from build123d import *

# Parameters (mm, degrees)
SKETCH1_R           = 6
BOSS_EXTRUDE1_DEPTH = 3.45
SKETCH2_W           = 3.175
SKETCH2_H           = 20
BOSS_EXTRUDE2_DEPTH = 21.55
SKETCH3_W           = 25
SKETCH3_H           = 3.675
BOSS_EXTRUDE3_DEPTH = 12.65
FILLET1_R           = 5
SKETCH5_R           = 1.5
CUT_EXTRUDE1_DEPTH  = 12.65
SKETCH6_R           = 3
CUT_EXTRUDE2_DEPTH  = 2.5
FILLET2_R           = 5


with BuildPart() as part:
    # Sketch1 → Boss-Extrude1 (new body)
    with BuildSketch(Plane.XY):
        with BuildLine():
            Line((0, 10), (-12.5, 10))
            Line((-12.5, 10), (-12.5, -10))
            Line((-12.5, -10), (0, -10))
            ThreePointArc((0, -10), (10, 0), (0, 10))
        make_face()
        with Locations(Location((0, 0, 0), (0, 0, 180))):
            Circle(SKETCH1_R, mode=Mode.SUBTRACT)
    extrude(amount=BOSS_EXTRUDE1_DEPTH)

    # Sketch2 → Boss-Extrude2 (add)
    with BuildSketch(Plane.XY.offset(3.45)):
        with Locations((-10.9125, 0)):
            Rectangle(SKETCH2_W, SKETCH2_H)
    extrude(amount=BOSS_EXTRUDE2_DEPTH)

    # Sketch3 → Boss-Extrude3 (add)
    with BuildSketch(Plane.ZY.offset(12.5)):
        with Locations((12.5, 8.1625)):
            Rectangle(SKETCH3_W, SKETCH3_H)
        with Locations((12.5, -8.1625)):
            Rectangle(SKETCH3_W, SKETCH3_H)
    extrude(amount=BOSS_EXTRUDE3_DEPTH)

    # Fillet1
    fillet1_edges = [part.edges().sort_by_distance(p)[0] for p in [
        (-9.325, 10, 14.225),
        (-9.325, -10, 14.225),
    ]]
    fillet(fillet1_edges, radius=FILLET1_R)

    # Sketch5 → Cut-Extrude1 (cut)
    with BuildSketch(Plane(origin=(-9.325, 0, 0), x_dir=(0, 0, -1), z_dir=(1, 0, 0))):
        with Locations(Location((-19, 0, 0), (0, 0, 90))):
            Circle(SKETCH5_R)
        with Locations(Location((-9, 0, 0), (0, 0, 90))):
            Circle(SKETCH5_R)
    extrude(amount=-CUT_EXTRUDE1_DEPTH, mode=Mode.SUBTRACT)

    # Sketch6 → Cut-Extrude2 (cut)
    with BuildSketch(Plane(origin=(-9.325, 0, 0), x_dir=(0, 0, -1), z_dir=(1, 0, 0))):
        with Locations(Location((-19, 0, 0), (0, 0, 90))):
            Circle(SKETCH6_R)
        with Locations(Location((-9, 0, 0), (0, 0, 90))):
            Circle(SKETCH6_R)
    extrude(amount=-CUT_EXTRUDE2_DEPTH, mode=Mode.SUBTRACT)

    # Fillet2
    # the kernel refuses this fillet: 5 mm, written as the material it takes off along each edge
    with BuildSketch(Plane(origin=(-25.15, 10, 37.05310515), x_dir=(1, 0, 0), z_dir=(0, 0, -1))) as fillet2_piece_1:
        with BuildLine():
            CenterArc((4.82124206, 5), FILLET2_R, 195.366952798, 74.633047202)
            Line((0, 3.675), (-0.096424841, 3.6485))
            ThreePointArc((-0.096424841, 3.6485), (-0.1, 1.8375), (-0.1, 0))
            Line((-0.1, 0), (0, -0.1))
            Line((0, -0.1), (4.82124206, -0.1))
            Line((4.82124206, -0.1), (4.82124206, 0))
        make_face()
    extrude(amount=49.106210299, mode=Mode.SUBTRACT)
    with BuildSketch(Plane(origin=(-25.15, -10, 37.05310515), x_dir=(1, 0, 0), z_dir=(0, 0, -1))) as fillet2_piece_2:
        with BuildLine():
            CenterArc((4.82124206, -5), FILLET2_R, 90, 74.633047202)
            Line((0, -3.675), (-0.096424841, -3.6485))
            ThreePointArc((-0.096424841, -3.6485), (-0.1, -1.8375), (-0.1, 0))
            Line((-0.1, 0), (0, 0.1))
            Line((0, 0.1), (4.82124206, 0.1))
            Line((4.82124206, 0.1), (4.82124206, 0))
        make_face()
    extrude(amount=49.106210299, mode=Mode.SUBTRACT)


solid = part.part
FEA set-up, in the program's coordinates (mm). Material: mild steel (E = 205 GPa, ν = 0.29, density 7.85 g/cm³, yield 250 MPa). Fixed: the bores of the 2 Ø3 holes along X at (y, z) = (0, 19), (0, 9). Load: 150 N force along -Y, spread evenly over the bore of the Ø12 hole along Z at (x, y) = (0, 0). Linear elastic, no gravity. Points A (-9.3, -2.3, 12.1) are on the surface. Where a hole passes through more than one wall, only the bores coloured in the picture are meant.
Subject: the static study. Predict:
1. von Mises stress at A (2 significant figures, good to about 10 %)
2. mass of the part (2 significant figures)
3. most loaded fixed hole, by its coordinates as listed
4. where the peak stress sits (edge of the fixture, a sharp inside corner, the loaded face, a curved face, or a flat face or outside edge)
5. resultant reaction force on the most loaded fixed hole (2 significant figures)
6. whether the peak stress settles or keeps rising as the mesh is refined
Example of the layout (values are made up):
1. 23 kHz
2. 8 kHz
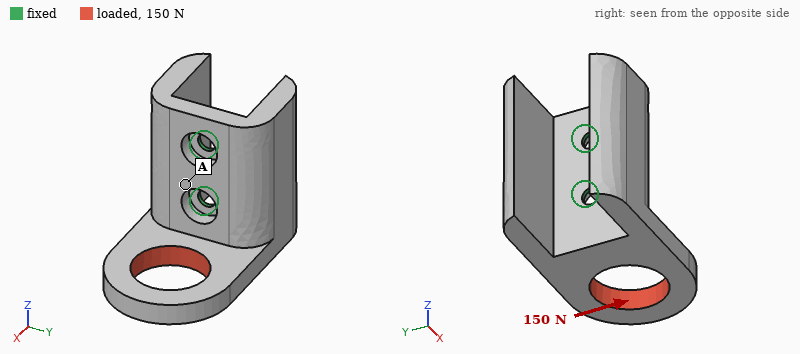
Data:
1. 45 MPa
2. 32 g
3. (0, 9)
4. edge of the fixture
5. 220 N
6. keeps rising
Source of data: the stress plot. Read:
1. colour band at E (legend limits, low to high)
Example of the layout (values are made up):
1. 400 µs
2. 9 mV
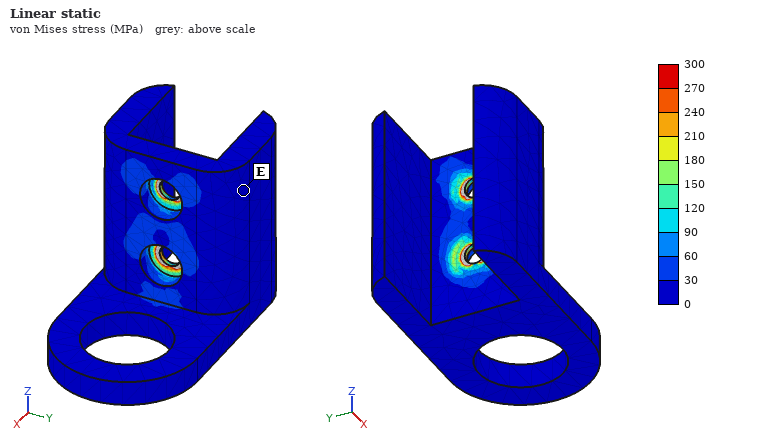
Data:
1. 0 to 30 MPa
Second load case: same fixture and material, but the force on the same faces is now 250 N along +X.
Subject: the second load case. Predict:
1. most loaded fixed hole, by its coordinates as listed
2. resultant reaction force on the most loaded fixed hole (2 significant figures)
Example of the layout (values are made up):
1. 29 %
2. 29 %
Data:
1. (0, 9)
2. 400 N
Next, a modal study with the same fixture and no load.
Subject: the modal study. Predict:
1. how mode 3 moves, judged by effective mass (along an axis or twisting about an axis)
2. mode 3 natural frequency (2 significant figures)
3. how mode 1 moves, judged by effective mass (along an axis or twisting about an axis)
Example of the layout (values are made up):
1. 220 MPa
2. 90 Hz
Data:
1. along Y
2. 7200 Hz
3. twisting about Z
